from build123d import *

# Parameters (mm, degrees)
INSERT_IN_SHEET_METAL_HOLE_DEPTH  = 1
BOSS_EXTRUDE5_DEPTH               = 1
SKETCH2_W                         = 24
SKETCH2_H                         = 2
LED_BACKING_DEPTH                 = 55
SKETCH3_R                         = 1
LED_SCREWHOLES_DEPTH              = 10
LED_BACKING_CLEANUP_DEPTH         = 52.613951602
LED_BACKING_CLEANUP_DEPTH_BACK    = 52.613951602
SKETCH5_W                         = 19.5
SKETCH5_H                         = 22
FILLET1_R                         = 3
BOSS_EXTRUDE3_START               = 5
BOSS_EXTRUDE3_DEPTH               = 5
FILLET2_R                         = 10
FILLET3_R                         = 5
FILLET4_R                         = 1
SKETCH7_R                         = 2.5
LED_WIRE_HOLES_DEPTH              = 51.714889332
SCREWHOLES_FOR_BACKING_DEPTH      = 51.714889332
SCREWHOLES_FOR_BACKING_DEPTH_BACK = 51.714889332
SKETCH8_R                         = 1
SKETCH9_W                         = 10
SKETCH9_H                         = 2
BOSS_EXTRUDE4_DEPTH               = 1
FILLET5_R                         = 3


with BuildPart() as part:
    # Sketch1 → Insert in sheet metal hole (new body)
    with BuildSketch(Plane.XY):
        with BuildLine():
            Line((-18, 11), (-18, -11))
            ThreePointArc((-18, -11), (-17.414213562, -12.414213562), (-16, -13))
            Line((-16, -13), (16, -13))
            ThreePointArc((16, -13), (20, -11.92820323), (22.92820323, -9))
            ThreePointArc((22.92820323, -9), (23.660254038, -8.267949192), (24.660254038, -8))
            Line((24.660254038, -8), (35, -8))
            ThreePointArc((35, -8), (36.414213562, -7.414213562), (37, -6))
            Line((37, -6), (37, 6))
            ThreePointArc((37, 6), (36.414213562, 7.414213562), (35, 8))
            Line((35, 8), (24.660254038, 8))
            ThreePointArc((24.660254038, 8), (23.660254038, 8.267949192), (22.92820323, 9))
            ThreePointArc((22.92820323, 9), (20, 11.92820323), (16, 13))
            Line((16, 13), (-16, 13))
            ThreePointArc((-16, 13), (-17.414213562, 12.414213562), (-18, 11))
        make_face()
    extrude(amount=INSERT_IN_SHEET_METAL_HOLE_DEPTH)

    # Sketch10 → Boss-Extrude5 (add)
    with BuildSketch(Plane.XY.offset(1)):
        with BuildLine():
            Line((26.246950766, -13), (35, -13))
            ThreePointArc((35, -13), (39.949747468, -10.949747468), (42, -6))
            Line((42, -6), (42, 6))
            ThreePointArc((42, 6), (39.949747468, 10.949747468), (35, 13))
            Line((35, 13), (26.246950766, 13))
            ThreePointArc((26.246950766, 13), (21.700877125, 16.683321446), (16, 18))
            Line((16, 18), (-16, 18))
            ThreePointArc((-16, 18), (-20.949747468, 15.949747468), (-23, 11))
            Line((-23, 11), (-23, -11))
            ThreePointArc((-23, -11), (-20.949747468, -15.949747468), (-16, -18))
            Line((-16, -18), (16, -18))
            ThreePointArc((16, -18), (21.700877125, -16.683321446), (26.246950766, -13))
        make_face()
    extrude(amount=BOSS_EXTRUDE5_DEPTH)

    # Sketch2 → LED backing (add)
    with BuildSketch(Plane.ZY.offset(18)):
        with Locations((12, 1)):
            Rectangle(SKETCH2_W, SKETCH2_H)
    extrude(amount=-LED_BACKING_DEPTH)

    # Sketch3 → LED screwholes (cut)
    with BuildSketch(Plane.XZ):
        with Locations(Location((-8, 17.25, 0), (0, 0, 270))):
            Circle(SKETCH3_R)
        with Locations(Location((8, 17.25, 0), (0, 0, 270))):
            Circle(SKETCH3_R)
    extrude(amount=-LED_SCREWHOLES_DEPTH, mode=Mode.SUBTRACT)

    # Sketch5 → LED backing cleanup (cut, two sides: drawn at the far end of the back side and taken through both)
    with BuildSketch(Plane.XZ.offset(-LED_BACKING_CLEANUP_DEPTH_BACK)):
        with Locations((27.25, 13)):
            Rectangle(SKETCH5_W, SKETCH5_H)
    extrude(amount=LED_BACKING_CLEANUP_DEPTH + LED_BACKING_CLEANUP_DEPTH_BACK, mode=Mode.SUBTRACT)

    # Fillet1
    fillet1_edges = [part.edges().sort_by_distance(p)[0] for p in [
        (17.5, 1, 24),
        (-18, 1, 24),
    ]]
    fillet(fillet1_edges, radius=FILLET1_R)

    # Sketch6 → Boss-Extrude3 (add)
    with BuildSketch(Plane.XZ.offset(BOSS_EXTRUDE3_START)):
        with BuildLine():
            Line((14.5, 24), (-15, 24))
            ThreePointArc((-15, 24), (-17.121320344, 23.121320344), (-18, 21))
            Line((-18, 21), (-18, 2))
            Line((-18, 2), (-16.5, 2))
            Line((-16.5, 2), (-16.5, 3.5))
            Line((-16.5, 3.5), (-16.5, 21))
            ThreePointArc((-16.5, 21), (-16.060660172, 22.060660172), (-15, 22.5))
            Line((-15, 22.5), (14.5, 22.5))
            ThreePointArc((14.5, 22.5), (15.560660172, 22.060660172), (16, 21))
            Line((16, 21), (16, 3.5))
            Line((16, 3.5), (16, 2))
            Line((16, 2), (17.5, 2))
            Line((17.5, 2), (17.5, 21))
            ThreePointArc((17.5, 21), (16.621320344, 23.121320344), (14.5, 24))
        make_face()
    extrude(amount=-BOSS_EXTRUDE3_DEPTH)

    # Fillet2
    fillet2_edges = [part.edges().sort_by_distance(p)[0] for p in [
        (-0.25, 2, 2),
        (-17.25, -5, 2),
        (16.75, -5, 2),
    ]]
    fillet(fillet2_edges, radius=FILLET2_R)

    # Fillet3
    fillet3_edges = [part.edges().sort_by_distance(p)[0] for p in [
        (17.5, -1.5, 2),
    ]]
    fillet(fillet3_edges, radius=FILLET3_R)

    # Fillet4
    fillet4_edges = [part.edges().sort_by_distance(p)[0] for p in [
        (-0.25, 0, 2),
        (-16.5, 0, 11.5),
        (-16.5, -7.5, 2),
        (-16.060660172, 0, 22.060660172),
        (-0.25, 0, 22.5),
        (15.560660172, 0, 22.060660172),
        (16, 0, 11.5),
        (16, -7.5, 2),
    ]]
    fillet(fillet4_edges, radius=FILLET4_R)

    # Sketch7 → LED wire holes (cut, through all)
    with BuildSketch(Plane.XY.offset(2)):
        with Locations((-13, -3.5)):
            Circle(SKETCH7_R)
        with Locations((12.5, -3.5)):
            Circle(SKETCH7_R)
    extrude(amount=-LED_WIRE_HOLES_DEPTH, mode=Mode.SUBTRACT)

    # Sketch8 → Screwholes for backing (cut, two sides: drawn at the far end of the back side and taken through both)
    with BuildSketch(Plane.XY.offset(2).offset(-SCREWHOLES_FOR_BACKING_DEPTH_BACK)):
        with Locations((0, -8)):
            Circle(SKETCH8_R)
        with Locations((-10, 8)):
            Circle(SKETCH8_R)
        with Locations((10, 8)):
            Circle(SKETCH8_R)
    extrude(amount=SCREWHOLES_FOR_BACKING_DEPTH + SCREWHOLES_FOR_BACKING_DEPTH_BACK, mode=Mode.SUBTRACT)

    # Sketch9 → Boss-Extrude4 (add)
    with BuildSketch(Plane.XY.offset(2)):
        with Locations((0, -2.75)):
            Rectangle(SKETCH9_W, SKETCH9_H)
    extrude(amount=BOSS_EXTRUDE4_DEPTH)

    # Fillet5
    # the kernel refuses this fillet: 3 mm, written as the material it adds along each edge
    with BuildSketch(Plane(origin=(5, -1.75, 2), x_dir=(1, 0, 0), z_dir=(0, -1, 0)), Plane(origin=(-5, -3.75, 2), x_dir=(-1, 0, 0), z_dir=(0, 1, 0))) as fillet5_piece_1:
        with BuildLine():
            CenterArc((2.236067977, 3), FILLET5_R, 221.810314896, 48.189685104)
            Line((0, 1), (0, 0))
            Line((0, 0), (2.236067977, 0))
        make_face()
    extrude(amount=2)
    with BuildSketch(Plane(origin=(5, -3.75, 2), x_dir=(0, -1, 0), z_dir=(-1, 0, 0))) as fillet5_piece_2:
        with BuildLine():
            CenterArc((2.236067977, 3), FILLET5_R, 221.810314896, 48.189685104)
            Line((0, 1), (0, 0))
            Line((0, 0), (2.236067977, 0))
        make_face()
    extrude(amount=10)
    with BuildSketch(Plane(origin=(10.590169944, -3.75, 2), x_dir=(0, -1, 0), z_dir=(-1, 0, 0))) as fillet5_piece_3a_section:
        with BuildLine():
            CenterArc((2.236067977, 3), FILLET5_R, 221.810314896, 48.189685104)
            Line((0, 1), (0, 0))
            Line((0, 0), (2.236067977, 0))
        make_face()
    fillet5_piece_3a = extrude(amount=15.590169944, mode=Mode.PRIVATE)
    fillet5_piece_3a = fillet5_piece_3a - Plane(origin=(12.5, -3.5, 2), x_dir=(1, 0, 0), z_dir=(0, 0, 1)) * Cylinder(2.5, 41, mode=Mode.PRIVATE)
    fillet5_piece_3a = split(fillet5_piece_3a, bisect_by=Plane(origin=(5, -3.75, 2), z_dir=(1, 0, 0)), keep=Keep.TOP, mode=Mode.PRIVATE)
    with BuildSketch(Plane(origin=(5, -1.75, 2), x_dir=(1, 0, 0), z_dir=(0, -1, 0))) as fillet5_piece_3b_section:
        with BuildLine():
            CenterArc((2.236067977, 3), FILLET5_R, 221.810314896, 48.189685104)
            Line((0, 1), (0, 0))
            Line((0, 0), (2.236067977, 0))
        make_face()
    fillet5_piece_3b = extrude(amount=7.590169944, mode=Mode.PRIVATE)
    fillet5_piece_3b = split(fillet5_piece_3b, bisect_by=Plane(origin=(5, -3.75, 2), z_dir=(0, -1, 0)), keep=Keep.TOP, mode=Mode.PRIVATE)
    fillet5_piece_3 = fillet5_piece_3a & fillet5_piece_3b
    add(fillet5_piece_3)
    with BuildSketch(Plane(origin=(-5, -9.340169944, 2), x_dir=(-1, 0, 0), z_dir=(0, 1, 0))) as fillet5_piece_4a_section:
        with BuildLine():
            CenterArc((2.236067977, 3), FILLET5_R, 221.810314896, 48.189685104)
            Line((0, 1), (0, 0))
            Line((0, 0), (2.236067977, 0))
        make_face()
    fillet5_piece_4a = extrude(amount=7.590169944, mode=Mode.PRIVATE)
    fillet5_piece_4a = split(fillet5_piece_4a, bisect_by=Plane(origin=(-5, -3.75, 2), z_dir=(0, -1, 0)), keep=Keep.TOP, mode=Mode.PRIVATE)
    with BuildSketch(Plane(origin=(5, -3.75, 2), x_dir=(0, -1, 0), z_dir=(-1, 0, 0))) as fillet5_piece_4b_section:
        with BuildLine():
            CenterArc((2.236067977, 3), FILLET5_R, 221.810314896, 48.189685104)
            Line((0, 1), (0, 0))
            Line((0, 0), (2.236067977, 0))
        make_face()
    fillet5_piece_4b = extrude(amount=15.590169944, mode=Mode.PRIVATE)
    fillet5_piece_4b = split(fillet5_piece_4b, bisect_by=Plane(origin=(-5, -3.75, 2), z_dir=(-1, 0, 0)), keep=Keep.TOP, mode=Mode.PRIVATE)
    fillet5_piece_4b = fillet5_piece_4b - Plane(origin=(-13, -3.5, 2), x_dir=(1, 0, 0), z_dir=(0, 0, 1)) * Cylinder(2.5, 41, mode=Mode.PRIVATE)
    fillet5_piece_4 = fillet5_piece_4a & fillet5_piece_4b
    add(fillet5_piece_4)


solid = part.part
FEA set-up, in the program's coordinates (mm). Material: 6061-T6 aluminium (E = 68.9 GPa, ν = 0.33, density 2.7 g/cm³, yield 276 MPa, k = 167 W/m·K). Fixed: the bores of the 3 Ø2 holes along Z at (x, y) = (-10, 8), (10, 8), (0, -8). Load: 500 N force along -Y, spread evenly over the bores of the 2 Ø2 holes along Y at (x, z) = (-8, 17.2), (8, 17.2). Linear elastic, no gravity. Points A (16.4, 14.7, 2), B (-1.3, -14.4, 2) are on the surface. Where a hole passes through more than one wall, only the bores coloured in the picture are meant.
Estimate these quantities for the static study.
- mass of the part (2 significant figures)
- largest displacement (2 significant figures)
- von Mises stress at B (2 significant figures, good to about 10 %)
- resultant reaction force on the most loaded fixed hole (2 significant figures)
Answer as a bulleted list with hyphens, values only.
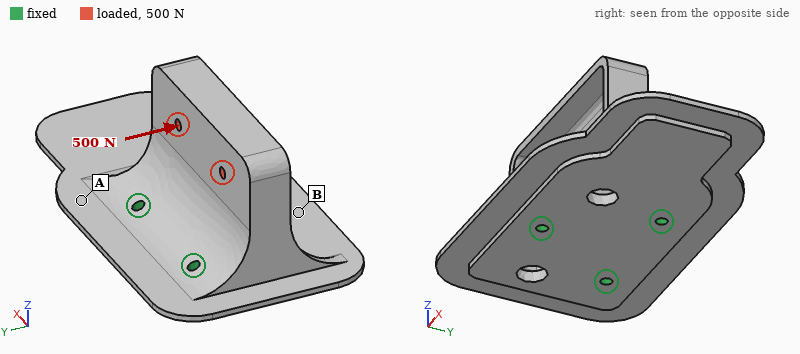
- 17 g
- 0.13 mm
- 39 MPa
- 340 N
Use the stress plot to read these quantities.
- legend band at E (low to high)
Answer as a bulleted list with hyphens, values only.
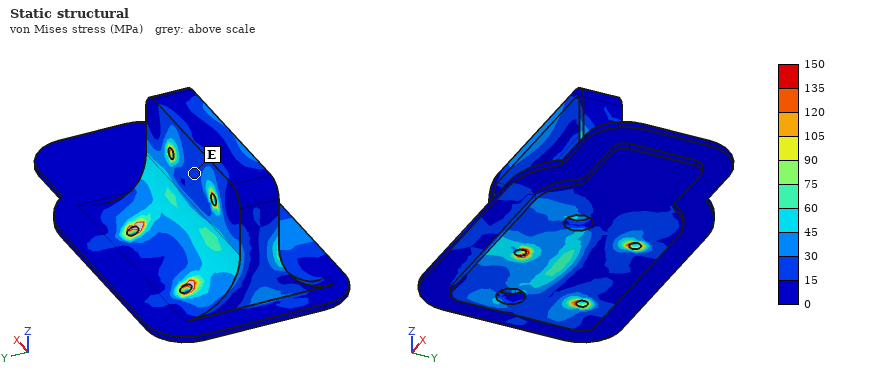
- 15 to 30 MPa
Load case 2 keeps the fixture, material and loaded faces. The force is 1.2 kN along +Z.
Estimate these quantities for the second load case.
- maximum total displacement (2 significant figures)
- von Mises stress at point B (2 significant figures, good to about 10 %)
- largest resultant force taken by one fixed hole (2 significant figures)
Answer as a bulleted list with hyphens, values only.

- 60 µm
- 28 MPa
- 440 N
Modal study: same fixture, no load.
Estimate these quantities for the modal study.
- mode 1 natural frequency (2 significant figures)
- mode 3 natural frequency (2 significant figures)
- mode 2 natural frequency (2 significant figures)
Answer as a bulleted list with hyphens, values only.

- 3300 Hz
- 5900 Hz
- 4900 Hz
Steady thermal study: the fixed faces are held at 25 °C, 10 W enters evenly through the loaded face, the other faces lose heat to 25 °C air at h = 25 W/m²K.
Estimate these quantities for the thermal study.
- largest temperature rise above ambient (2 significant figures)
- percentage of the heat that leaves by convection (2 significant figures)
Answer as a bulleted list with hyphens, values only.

- 14 K
- 6.9 %
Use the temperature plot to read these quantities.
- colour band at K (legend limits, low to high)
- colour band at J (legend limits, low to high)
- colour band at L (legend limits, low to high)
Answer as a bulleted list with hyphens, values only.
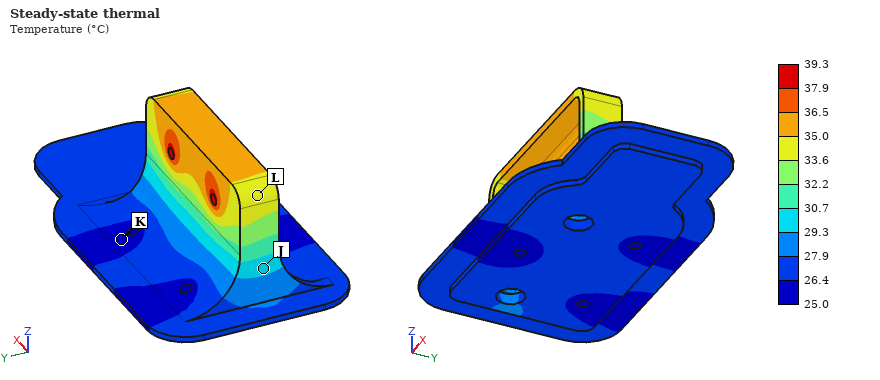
- 25.0 to 26.4 °C
- 29.3 to 30.7 °C
- 33.6 to 35.0 °C
